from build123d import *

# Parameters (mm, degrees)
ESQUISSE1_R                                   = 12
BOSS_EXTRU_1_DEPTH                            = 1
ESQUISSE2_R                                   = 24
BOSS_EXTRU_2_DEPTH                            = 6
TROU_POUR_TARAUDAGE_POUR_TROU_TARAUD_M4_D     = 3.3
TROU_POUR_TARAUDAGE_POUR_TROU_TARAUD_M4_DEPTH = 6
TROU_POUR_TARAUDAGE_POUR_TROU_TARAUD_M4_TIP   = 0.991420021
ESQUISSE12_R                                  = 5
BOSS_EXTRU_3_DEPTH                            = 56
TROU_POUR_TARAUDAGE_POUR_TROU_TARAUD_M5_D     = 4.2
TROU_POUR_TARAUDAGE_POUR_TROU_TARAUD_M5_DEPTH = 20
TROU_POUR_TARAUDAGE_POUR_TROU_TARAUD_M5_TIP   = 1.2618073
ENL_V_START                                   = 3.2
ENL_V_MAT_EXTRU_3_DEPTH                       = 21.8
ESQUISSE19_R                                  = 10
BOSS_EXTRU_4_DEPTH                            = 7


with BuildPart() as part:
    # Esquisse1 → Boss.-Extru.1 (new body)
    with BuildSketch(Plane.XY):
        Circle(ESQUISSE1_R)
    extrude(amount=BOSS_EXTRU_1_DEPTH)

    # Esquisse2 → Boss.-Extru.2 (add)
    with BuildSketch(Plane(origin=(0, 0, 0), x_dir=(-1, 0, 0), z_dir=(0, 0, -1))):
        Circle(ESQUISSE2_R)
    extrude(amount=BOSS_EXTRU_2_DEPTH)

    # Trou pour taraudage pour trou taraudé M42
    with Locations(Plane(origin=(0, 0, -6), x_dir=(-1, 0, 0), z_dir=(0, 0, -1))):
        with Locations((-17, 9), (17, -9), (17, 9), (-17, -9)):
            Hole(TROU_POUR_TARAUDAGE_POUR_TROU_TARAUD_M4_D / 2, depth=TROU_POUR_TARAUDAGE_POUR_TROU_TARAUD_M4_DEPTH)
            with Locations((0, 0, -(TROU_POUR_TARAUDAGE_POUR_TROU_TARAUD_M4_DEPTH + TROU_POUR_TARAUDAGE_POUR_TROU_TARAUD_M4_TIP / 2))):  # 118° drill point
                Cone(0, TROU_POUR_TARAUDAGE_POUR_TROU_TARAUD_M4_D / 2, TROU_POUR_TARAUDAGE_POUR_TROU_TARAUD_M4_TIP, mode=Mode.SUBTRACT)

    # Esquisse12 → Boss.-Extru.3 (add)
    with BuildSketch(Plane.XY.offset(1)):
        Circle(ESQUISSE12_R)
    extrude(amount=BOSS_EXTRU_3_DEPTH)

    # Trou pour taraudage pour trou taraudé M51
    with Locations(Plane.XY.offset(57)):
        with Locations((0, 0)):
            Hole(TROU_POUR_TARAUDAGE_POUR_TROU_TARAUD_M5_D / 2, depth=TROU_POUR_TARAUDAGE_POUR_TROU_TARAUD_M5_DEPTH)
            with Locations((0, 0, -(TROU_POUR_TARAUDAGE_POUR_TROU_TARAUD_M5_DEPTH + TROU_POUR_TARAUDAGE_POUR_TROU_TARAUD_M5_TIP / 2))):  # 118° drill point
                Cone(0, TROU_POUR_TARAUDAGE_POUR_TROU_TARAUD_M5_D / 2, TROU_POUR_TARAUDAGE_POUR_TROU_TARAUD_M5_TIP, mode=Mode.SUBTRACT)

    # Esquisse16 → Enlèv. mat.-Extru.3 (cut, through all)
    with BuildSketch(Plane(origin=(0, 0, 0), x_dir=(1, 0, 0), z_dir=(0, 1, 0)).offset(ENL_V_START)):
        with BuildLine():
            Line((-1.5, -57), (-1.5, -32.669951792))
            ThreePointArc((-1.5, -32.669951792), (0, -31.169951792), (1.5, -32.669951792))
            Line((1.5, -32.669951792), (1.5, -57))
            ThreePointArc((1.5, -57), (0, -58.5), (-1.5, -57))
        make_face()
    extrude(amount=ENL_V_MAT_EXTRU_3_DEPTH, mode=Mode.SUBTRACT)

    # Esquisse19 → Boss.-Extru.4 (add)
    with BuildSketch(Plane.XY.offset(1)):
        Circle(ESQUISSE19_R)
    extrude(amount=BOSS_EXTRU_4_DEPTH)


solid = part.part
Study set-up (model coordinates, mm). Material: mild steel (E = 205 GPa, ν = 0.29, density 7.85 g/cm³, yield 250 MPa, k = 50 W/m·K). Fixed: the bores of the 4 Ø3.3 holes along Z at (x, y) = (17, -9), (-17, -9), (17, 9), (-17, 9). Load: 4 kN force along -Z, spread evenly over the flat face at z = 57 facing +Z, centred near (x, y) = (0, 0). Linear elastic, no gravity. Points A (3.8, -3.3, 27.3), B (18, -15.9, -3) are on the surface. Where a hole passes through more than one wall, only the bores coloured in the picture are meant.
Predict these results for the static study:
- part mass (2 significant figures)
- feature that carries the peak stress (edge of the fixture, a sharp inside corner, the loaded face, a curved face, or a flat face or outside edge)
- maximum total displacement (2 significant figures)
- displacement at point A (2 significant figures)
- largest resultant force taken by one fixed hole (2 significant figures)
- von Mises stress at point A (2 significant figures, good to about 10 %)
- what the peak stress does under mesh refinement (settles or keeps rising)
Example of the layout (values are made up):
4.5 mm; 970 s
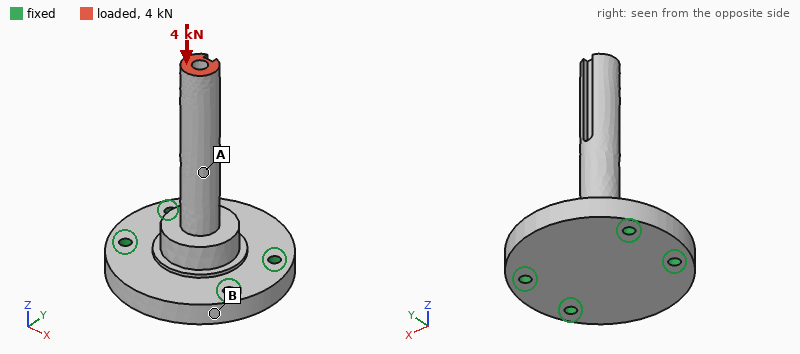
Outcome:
130 g; edge of the fixture; 26 µm; 12 µm; 1.1 kN; 60 MPa; keeps rising
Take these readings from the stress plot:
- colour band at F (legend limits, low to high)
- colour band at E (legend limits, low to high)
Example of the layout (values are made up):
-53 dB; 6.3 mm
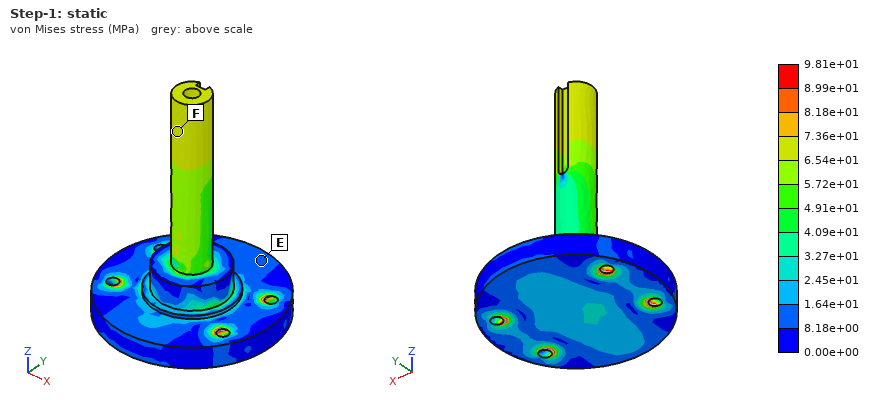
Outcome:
6.54e+01 to 7.36e+01 MPa; 8.18e+00 to 1.64e+01 MPa
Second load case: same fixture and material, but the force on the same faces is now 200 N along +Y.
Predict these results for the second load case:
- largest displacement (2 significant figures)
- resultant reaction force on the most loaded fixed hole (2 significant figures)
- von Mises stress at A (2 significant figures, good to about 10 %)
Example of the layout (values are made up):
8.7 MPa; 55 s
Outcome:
0.10 mm; 290 N; 40 MPa
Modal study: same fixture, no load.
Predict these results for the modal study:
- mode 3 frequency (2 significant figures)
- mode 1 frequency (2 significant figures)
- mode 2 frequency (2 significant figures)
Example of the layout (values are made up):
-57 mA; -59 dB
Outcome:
12 kHz; 2800 Hz; 2900 Hz
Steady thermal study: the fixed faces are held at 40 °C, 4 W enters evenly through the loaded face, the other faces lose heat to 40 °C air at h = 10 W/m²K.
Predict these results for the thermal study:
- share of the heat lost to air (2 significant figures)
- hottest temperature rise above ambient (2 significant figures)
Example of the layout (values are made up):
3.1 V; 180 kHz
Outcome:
16 %; 57 K
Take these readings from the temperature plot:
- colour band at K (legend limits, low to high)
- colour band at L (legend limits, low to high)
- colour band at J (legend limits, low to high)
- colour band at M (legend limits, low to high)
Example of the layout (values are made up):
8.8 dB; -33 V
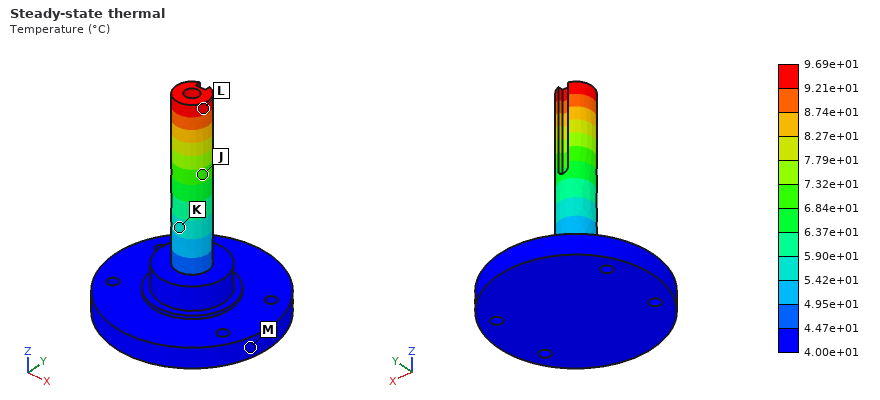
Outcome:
5.42e+01 to 5.90e+01 °C; 9.21e+01 to 9.69e+01 °C; 6.84e+01 to 7.32e+01 °C; 4.00e+01 to 4.47e+01 °C
